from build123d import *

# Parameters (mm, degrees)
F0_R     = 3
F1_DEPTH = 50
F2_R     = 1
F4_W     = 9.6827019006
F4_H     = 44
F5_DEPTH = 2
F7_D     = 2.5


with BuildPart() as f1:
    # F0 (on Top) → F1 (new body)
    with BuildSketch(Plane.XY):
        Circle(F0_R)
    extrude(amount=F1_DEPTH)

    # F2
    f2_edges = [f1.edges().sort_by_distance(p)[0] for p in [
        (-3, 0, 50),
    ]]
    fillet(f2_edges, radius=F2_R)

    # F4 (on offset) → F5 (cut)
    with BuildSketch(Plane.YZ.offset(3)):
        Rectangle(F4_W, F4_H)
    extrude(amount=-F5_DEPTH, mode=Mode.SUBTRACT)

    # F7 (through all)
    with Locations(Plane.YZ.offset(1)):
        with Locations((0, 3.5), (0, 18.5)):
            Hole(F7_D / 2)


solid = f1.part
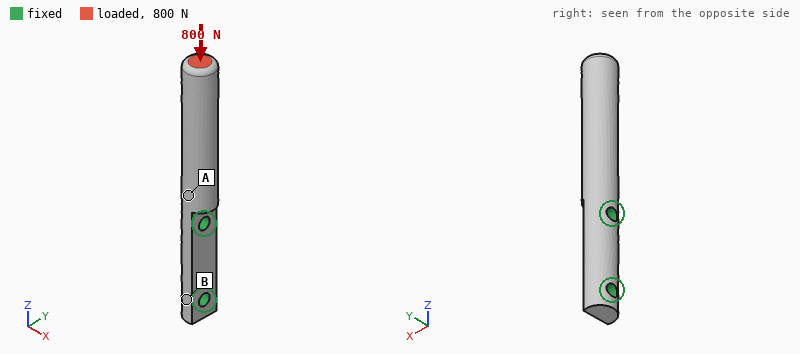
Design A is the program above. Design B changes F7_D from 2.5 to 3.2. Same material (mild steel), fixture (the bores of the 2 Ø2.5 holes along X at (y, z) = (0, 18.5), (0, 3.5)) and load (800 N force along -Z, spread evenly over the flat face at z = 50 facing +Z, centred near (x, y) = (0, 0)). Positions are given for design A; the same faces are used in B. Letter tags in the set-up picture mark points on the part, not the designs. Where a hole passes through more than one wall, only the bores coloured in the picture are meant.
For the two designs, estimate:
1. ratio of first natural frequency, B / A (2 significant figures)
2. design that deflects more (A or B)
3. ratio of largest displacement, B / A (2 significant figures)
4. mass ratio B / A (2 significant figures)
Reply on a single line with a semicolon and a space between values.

1.0; A; 0.89; 0.98
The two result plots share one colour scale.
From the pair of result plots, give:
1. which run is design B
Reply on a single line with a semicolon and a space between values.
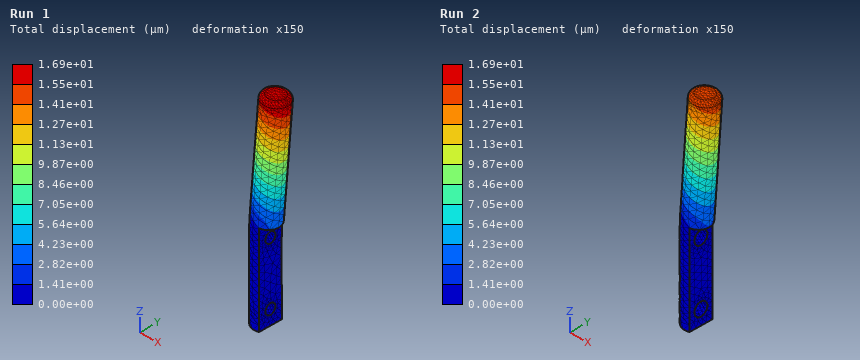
Run 2
